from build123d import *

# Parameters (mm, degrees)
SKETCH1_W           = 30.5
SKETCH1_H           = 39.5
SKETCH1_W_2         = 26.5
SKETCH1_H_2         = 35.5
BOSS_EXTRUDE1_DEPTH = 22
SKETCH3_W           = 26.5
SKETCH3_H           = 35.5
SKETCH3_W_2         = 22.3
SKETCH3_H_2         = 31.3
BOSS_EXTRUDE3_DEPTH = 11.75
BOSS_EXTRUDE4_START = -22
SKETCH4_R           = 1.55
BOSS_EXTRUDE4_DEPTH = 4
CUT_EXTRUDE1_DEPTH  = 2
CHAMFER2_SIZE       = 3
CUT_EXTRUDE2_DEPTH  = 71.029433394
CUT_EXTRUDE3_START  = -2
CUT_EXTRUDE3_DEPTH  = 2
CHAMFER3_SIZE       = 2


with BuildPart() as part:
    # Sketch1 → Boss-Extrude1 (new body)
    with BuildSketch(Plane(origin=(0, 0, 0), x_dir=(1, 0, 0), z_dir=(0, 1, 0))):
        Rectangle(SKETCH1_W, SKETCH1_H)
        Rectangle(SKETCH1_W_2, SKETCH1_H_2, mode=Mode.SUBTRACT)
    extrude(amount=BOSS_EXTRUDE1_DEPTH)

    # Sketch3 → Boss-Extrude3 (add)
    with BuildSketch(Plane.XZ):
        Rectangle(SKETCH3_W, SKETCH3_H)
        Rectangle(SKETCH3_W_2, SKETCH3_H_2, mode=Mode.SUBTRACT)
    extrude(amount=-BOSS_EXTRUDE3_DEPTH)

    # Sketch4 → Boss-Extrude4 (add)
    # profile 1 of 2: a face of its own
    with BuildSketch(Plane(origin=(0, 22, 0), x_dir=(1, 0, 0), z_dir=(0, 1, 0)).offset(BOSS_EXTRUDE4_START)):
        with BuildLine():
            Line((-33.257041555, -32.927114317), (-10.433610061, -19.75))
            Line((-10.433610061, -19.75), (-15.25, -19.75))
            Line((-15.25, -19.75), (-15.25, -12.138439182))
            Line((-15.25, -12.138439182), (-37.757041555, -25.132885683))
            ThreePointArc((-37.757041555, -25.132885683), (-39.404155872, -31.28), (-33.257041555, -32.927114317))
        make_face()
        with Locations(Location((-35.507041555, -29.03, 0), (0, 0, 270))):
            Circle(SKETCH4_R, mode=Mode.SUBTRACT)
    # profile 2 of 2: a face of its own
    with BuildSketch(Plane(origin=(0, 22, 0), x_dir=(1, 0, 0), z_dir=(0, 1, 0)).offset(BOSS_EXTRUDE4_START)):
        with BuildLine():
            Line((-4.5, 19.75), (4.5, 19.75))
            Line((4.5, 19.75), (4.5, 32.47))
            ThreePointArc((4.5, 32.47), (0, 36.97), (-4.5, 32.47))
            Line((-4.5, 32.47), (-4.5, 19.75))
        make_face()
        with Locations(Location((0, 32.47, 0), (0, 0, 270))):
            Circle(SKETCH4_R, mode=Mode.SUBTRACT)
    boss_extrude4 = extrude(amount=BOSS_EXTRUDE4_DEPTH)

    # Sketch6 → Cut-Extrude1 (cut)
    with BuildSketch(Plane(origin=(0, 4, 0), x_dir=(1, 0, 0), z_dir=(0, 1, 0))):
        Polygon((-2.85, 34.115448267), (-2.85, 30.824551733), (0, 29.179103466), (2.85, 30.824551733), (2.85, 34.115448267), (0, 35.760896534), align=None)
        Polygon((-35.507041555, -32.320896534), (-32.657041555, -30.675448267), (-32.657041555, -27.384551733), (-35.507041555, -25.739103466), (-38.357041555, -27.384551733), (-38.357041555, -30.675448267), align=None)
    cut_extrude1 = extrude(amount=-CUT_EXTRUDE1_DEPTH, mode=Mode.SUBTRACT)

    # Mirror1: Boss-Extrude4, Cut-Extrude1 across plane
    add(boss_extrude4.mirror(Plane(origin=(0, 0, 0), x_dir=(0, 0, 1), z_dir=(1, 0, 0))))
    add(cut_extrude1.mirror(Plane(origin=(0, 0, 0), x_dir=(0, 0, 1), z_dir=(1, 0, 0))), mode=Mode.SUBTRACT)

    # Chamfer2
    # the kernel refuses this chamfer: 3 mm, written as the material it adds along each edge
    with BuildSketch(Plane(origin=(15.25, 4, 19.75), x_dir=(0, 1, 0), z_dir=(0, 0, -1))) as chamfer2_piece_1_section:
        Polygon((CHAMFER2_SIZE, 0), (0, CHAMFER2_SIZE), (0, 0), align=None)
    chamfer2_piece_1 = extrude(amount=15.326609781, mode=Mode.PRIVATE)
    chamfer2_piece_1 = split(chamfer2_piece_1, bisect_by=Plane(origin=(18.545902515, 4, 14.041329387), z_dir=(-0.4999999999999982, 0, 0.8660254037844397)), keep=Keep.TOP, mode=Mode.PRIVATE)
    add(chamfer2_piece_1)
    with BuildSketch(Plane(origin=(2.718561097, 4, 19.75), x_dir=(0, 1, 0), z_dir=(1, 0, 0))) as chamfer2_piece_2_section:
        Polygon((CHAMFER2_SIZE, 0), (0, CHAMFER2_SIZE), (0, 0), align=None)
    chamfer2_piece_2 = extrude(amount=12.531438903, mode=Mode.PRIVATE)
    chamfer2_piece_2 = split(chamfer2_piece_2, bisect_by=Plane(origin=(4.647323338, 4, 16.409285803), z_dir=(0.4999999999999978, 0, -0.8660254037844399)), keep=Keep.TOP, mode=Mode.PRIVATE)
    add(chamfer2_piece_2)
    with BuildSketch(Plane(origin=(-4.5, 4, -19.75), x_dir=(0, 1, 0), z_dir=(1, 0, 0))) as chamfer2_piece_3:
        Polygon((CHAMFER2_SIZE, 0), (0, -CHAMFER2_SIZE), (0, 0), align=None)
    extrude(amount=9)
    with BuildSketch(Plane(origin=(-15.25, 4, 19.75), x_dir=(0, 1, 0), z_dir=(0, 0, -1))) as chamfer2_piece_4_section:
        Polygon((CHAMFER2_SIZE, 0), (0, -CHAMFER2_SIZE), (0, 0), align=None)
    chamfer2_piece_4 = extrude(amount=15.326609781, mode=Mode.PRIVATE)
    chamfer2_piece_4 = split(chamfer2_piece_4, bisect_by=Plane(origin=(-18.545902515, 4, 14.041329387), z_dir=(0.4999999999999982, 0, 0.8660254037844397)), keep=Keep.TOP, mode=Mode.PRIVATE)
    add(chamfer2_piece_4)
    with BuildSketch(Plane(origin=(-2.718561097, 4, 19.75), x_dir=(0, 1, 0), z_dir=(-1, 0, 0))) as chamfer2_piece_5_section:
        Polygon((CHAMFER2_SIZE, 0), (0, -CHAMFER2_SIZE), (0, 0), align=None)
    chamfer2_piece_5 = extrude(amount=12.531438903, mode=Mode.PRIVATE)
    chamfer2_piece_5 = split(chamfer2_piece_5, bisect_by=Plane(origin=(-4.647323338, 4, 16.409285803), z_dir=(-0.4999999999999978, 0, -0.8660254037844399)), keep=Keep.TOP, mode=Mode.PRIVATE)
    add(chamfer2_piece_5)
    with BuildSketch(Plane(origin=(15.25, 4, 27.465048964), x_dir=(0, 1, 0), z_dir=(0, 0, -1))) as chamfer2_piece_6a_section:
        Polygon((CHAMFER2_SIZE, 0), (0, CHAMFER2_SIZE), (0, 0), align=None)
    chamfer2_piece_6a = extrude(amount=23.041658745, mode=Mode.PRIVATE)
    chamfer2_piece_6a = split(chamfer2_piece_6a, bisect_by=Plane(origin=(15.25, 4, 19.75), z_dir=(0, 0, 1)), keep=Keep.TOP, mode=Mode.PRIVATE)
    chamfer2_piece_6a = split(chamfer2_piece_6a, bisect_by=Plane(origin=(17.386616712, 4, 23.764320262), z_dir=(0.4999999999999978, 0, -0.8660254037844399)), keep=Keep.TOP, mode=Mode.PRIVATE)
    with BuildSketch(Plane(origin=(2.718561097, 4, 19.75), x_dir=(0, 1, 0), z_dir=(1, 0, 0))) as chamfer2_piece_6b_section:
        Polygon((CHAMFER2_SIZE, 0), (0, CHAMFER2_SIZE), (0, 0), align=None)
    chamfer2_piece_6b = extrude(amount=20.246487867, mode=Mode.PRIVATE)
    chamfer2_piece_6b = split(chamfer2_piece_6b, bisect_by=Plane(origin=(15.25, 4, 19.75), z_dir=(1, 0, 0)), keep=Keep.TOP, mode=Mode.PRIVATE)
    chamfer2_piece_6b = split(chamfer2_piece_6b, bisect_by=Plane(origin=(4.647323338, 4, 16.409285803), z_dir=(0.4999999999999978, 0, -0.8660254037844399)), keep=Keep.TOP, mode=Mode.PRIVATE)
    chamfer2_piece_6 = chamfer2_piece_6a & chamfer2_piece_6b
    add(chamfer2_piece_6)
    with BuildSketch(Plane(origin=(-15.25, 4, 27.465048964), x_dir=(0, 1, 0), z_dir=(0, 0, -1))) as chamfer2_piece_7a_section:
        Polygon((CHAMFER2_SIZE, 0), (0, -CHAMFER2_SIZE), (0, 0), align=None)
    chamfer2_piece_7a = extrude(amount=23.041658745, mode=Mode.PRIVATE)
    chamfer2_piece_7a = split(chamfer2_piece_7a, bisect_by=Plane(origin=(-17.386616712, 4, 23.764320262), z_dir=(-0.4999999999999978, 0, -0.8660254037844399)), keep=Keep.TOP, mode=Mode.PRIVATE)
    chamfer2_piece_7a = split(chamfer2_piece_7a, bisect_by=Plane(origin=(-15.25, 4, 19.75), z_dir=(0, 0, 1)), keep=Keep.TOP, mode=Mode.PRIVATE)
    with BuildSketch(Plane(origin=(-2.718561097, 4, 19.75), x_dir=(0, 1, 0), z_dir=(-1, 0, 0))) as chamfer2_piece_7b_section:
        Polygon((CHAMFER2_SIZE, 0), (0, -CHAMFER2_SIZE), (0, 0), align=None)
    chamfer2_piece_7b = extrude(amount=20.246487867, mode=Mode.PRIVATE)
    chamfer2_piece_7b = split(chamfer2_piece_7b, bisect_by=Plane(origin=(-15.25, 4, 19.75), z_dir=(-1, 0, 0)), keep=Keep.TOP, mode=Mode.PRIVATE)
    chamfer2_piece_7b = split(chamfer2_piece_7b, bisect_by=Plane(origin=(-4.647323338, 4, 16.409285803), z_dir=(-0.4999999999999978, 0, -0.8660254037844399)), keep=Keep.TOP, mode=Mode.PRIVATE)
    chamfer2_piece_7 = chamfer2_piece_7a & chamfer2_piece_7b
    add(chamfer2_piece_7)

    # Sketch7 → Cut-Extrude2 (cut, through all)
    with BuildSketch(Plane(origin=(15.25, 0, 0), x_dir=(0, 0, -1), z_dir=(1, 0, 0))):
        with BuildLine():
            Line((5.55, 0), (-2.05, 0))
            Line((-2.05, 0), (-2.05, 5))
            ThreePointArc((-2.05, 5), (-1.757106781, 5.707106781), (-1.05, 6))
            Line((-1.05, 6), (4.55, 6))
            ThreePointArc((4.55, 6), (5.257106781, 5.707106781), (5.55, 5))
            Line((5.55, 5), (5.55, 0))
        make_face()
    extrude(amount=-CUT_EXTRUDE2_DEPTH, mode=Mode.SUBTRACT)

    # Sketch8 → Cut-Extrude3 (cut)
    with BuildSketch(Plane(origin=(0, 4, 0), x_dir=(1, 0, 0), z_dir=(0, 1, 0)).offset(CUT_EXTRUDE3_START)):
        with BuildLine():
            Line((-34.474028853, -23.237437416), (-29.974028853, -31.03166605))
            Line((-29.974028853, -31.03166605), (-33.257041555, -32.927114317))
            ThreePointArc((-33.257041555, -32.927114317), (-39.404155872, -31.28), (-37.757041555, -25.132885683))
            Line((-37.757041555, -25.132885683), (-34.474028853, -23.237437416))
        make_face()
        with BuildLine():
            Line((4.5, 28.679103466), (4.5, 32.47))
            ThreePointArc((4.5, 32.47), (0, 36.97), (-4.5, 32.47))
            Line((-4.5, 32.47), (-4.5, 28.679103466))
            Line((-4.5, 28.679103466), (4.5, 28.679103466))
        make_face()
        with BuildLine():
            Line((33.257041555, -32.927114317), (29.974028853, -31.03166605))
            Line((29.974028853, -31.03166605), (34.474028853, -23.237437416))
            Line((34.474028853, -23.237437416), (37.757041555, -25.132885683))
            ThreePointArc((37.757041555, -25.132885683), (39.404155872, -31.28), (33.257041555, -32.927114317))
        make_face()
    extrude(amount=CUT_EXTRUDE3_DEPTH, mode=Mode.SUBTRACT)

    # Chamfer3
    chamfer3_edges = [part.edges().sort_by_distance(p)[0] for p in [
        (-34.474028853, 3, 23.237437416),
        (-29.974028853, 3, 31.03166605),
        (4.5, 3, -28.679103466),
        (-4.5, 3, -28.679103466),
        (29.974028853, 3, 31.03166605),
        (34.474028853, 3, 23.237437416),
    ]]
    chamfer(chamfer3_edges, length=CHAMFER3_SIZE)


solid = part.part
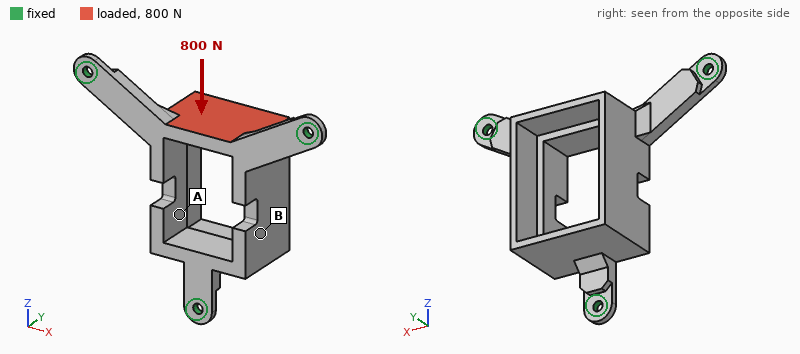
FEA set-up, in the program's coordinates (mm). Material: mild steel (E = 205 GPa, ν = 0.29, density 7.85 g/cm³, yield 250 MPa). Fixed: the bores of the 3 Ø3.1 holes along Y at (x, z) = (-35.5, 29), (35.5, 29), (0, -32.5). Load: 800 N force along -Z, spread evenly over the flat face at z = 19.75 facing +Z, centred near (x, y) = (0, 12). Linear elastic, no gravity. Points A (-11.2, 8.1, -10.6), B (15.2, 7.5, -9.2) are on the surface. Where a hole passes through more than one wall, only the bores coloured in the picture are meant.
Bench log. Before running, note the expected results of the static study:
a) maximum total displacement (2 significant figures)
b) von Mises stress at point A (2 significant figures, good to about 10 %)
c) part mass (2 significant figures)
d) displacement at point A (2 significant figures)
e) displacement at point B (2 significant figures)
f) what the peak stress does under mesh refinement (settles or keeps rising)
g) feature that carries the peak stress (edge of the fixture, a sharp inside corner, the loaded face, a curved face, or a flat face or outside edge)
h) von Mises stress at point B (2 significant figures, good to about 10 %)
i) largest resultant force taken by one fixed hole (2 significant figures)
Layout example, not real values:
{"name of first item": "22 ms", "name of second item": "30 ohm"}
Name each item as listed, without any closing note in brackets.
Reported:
{"maximum total displacement": "29 µm", "von Mises stress at point A": "16 MPa", "part mass": "83 g", "displacement at point A": "7.0 µm", "displacement at point B": "8.6 µm", "what the peak stress does under mesh refinement": "keeps rising", "feature that carries the peak stress": "edge of the fixture", "von Mises stress at point B": "6.8 MPa", "largest resultant force taken by one fixed hole": "500 N"}
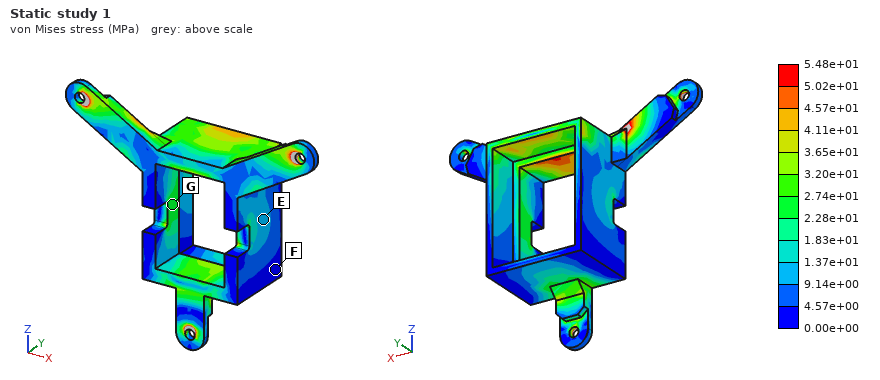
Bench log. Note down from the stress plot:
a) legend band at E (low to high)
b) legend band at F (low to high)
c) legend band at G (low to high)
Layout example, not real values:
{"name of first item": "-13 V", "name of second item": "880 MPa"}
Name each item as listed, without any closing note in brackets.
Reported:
{"legend band at E": "9.14e+00 to 1.37e+01 MPa", "legend band at F": "0.00e+00 to 4.57e+00 MPa", "legend band at G": "2.28e+01 to 2.74e+01 MPa"}
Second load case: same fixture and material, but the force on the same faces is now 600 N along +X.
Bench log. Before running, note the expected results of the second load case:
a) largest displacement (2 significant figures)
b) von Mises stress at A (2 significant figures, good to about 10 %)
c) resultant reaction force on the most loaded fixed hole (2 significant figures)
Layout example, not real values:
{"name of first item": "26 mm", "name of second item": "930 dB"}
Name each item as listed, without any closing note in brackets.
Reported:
{"largest displacement": "16 µm", "von Mises stress at A": "8.4 MPa", "resultant reaction force on the most loaded fixed hole": "350 N"}
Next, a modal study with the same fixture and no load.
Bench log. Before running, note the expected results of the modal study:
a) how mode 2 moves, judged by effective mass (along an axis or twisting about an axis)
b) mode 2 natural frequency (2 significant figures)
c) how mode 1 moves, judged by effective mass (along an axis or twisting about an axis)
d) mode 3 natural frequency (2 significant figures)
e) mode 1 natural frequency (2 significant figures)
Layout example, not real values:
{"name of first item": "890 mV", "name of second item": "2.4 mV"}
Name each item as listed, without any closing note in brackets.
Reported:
{"how mode 2 moves, judged by effective mass": "along Y", "mode 2 natural frequency": "3000 Hz", "how mode 1 moves, judged by effective mass": "along X", "mode 3 natural frequency": "5500 Hz", "mode 1 natural frequency": "2800 Hz"}
